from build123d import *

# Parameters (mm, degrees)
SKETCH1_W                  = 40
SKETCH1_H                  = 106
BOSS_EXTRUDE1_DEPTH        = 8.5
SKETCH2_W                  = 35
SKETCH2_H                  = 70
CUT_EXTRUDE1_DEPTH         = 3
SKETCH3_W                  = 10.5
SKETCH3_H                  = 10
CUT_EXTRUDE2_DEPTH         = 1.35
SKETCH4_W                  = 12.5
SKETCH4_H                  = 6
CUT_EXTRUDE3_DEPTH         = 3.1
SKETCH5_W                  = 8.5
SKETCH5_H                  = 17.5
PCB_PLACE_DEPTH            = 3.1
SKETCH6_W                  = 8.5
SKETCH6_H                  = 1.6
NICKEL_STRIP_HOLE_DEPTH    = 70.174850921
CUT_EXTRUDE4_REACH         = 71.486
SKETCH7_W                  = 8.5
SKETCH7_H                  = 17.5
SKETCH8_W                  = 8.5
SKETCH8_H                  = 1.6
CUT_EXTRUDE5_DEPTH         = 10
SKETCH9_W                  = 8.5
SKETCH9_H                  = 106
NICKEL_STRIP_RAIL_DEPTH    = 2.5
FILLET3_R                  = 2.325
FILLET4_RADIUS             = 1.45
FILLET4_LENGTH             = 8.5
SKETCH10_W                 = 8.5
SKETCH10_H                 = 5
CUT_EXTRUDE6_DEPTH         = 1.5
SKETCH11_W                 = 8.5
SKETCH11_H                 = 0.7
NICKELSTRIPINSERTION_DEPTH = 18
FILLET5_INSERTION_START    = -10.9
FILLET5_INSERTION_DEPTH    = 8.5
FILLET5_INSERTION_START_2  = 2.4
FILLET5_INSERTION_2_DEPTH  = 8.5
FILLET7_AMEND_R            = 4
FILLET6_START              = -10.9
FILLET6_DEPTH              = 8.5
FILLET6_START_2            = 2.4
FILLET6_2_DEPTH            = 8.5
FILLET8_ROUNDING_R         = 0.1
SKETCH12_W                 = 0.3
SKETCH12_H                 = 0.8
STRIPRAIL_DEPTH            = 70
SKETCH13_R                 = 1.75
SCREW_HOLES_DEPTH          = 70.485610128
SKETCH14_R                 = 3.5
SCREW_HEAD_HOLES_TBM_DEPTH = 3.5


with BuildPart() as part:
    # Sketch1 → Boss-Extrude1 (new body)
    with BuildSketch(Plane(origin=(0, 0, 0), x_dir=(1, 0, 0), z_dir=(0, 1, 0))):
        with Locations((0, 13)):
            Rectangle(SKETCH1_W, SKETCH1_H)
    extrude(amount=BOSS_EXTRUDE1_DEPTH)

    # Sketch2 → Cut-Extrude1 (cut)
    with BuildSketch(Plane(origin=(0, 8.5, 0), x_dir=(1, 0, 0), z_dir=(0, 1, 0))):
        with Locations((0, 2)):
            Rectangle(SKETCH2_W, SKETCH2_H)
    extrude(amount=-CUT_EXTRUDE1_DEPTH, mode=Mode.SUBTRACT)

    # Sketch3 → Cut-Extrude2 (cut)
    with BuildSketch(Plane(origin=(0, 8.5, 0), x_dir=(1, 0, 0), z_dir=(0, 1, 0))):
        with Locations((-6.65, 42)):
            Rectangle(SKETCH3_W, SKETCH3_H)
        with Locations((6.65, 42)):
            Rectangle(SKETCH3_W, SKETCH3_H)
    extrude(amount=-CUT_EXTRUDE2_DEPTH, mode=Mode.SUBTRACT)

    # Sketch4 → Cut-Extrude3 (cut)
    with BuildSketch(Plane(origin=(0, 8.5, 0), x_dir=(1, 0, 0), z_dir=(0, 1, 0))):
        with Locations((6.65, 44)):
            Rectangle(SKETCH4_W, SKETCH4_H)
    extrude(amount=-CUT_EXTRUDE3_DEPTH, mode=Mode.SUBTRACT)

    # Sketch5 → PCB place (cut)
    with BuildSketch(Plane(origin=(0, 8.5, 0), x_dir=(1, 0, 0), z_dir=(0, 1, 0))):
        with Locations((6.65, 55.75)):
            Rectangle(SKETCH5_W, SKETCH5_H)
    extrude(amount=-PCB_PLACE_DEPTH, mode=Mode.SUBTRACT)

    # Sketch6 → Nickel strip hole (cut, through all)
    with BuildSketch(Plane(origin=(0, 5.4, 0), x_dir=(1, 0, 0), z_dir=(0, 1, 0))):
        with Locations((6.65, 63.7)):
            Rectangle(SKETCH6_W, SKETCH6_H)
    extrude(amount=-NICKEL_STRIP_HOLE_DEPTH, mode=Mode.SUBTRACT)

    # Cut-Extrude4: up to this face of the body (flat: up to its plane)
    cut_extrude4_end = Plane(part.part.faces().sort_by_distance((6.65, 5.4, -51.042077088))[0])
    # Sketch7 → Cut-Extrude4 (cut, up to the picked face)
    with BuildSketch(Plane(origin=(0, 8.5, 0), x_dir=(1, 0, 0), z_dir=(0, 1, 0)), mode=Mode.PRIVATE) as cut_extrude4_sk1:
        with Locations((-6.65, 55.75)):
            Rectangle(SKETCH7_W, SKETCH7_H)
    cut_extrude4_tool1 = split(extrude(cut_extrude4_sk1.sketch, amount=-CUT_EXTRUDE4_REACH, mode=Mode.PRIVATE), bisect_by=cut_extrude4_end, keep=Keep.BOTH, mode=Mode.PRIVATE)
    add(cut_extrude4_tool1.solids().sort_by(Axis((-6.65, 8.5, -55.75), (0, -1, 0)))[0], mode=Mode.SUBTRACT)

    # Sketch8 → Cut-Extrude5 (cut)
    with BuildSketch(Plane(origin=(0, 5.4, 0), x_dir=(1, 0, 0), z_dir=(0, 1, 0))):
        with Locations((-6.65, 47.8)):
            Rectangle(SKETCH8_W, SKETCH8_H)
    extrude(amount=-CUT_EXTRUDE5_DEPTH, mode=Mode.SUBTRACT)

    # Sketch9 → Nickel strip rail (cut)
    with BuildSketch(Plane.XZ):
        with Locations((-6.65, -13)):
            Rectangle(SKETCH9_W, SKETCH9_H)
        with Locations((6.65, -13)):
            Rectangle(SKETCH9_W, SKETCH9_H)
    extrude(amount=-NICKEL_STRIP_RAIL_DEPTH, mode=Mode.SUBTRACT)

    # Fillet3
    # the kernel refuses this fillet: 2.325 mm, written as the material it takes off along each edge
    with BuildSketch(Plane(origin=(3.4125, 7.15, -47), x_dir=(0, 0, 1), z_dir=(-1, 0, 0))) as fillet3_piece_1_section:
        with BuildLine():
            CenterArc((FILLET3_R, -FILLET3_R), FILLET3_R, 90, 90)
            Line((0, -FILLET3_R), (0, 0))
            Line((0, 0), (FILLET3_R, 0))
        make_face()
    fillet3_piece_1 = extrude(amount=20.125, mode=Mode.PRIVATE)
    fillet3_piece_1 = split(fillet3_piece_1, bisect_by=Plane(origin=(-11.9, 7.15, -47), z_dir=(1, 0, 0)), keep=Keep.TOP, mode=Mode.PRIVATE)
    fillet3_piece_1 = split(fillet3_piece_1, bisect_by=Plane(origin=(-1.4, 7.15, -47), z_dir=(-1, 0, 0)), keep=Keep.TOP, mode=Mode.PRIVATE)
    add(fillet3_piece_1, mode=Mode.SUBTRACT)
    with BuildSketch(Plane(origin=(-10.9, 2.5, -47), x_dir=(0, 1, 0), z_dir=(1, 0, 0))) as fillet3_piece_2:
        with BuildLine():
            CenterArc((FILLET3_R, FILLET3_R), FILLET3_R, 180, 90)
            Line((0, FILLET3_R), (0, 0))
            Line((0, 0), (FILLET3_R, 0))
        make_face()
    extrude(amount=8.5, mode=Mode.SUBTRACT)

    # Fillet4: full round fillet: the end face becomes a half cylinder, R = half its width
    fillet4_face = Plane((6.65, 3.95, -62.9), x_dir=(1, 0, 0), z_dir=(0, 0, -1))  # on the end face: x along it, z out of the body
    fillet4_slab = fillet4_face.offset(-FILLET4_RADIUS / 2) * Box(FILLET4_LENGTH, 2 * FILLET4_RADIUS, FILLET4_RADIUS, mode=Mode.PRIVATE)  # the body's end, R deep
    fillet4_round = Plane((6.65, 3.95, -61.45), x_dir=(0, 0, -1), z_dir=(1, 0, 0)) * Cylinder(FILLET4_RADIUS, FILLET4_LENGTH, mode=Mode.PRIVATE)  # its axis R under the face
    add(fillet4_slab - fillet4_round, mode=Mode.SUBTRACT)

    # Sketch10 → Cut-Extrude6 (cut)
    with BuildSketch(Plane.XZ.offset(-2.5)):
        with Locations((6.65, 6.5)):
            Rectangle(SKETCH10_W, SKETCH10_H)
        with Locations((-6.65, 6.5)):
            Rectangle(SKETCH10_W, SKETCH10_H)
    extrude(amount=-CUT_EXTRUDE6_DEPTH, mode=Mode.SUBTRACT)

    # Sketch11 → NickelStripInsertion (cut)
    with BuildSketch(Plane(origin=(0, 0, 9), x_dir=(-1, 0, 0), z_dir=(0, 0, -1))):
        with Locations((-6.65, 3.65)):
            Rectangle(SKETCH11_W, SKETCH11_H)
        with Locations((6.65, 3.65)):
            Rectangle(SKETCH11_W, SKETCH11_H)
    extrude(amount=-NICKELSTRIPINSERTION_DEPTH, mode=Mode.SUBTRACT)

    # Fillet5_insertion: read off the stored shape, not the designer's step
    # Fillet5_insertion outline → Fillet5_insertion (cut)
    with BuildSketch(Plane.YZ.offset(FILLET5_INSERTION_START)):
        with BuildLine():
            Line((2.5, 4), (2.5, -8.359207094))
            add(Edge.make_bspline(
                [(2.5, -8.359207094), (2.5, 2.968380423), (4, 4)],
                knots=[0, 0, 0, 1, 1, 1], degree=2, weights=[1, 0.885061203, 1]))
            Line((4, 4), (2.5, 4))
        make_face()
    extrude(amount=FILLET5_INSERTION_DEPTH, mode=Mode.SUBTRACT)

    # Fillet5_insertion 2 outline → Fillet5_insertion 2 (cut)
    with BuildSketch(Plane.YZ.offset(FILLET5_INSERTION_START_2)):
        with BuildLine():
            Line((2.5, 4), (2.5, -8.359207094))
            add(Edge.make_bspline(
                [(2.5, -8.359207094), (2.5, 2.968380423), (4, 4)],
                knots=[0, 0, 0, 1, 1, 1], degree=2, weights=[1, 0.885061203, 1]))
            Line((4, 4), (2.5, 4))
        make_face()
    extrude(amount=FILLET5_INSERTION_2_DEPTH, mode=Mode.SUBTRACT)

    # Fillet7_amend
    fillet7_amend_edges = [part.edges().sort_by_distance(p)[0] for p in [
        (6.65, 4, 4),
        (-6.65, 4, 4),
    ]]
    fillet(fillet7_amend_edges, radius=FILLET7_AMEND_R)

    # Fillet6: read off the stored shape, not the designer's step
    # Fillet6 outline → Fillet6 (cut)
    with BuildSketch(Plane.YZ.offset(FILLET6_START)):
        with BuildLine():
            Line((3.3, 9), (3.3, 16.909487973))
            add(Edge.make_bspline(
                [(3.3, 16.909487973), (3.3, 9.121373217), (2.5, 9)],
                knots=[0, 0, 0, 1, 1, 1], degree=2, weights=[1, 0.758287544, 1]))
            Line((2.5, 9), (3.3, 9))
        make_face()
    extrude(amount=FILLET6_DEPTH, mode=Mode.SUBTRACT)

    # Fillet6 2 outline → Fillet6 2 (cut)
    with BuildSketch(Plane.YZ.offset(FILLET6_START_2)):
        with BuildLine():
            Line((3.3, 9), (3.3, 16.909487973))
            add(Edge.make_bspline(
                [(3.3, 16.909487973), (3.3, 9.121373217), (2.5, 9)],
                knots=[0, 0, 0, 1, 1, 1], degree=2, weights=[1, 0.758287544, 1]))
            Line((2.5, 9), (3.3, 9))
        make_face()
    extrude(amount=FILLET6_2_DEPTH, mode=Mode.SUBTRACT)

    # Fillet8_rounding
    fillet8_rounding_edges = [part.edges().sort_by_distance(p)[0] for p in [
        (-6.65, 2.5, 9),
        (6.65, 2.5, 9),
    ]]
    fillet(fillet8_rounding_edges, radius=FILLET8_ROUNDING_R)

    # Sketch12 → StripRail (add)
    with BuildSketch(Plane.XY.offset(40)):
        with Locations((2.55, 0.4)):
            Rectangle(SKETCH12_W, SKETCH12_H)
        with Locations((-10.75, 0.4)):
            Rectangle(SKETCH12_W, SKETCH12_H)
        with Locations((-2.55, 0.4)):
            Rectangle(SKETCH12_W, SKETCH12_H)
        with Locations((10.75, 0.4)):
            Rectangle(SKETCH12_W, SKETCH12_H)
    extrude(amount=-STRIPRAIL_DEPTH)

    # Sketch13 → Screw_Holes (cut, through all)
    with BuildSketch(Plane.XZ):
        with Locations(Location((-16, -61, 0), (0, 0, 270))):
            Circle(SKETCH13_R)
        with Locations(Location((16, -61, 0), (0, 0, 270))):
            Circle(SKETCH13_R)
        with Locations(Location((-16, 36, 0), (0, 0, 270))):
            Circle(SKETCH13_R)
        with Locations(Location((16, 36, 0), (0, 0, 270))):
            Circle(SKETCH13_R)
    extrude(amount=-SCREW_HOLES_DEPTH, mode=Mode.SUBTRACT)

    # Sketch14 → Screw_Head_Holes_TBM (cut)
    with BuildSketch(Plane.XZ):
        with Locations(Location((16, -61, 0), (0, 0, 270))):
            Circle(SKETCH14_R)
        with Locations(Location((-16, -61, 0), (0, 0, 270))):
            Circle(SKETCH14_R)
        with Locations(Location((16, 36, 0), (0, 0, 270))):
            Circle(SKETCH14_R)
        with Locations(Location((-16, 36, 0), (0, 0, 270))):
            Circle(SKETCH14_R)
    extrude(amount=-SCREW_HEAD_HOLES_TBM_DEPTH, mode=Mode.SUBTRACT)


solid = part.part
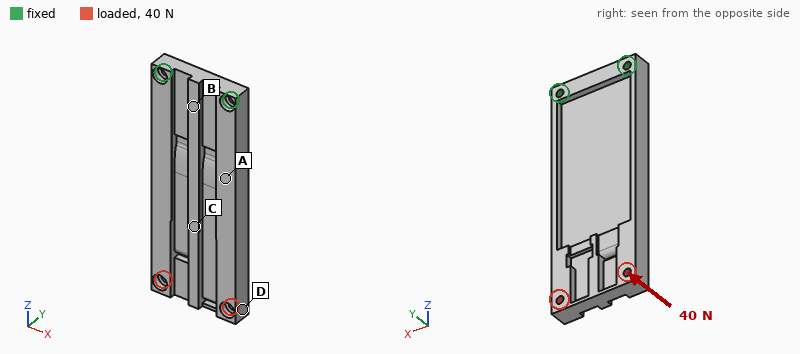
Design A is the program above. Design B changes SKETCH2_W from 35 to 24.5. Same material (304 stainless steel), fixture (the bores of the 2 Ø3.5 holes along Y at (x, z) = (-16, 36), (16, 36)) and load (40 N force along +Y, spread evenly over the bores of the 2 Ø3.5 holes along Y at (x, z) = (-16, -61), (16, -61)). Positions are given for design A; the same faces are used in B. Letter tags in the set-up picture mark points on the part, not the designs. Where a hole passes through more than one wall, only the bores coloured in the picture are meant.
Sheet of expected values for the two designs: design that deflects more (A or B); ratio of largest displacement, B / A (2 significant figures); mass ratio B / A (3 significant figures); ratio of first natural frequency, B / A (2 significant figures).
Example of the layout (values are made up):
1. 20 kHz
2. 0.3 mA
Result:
1. A
2. 0.64
3. 1.10
4. 1.2
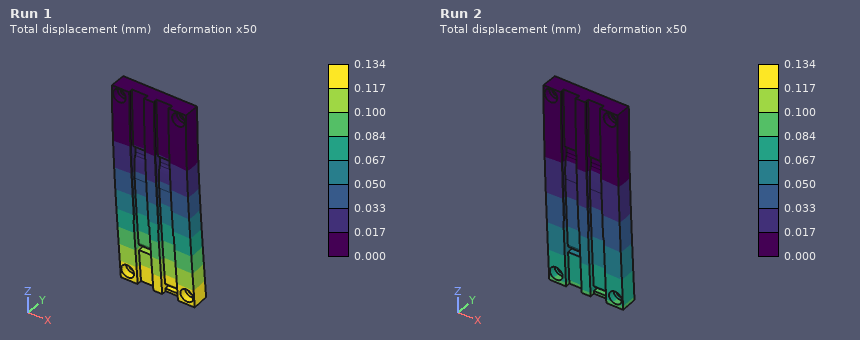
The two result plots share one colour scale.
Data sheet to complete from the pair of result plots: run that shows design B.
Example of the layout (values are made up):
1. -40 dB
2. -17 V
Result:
1. Run 2
